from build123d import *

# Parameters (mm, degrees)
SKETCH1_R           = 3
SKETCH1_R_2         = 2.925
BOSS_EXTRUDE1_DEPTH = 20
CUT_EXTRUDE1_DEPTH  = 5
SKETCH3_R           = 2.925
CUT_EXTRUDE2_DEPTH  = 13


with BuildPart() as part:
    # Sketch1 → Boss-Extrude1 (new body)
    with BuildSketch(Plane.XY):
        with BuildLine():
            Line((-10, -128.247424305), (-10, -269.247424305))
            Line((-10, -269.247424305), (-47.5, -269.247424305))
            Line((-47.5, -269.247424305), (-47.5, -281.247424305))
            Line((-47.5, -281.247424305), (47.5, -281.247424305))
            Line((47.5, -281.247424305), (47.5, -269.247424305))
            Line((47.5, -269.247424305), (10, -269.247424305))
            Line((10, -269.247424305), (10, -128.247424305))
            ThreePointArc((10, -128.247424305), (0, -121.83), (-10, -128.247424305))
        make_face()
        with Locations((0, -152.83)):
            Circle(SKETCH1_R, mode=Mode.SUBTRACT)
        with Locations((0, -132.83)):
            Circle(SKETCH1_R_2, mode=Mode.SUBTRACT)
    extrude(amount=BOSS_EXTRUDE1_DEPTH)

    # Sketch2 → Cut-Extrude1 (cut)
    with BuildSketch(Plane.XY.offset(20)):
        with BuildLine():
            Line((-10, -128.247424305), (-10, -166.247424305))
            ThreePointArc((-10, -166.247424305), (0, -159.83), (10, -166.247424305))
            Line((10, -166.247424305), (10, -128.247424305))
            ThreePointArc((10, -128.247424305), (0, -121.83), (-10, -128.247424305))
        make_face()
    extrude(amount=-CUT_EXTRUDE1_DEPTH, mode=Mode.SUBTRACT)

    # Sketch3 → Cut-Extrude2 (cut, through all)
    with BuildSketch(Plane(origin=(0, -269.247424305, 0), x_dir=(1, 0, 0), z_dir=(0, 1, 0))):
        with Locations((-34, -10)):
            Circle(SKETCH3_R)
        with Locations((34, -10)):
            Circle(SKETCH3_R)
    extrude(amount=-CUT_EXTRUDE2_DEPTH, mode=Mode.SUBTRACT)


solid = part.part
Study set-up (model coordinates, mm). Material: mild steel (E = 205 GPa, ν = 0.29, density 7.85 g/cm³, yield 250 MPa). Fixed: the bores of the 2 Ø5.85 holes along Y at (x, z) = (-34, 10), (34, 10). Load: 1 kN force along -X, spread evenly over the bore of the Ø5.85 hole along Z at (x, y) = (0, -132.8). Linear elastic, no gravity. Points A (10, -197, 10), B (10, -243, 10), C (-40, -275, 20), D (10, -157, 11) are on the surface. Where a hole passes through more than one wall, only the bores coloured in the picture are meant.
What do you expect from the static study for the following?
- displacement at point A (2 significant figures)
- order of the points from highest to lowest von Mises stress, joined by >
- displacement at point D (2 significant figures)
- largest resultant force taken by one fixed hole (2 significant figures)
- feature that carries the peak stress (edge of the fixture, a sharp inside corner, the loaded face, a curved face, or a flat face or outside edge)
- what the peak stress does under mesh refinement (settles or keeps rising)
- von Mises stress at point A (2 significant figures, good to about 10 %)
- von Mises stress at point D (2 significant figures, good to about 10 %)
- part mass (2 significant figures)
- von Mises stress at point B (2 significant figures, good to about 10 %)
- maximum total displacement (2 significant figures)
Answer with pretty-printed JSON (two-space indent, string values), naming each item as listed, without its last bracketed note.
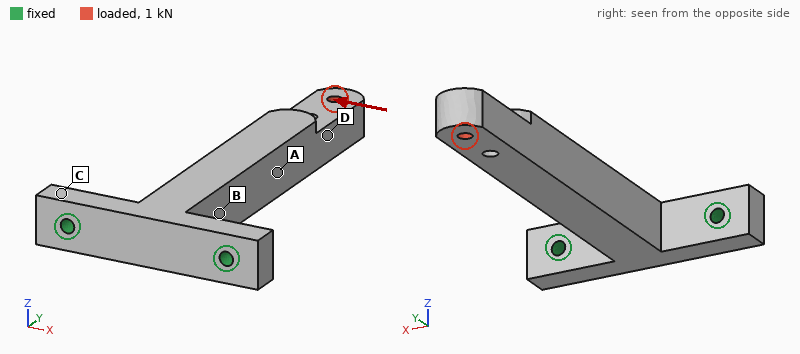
{
  "displacement at point A": "0.17 mm",
  "order of the points from highest to lowest von Mises stress, joined by >": "B > A > D > C",
  "displacement at point D": "0.32 mm",
  "largest resultant force taken by one fixed hole": "3.0 kN",
  "feature that carries the peak stress": "edge of the fixture",
  "what the peak stress does under mesh refinement": "keeps rising",
  "von Mises stress at point A": "48 MPa",
  "von Mises stress at point D": "29 MPa",
  "part mass": "590 g",
  "von Mises stress at point B": "83 MPa",
  "maximum total displacement": "0.48 mm"
}
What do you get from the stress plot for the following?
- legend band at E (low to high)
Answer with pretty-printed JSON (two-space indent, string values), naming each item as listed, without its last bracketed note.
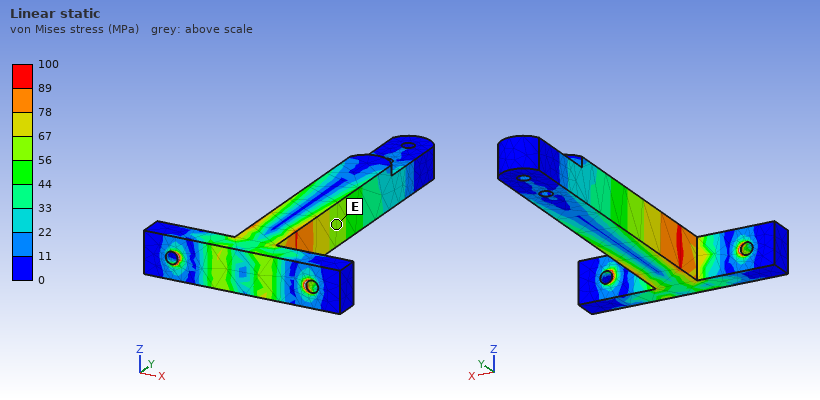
{
  "legend band at E": "56 to 67 MPa"
}
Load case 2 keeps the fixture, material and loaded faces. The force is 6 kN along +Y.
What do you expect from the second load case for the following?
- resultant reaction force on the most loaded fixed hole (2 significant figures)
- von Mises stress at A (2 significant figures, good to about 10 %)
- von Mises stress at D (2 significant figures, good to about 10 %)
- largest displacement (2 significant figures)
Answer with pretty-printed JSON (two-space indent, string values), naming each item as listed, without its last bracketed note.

{
  "resultant reaction force on the most loaded fixed hole": "3.1 kN",
  "von Mises stress at A": "15 MPa",
  "von Mises stress at D": "22 MPa",
  "largest displacement": "0.11 mm"
}
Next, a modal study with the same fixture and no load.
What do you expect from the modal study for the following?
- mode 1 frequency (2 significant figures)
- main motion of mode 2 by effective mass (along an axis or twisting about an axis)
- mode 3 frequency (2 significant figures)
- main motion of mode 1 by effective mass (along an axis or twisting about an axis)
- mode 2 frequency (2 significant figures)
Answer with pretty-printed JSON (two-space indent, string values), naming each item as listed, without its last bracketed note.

{
  "mode 1 frequency": "500 Hz",
  "main motion of mode 2 by effective mass": "along X",
  "mode 3 frequency": "3300 Hz",
  "main motion of mode 1 by effective mass": "along Z",
  "mode 2 frequency": "720 Hz"
}
